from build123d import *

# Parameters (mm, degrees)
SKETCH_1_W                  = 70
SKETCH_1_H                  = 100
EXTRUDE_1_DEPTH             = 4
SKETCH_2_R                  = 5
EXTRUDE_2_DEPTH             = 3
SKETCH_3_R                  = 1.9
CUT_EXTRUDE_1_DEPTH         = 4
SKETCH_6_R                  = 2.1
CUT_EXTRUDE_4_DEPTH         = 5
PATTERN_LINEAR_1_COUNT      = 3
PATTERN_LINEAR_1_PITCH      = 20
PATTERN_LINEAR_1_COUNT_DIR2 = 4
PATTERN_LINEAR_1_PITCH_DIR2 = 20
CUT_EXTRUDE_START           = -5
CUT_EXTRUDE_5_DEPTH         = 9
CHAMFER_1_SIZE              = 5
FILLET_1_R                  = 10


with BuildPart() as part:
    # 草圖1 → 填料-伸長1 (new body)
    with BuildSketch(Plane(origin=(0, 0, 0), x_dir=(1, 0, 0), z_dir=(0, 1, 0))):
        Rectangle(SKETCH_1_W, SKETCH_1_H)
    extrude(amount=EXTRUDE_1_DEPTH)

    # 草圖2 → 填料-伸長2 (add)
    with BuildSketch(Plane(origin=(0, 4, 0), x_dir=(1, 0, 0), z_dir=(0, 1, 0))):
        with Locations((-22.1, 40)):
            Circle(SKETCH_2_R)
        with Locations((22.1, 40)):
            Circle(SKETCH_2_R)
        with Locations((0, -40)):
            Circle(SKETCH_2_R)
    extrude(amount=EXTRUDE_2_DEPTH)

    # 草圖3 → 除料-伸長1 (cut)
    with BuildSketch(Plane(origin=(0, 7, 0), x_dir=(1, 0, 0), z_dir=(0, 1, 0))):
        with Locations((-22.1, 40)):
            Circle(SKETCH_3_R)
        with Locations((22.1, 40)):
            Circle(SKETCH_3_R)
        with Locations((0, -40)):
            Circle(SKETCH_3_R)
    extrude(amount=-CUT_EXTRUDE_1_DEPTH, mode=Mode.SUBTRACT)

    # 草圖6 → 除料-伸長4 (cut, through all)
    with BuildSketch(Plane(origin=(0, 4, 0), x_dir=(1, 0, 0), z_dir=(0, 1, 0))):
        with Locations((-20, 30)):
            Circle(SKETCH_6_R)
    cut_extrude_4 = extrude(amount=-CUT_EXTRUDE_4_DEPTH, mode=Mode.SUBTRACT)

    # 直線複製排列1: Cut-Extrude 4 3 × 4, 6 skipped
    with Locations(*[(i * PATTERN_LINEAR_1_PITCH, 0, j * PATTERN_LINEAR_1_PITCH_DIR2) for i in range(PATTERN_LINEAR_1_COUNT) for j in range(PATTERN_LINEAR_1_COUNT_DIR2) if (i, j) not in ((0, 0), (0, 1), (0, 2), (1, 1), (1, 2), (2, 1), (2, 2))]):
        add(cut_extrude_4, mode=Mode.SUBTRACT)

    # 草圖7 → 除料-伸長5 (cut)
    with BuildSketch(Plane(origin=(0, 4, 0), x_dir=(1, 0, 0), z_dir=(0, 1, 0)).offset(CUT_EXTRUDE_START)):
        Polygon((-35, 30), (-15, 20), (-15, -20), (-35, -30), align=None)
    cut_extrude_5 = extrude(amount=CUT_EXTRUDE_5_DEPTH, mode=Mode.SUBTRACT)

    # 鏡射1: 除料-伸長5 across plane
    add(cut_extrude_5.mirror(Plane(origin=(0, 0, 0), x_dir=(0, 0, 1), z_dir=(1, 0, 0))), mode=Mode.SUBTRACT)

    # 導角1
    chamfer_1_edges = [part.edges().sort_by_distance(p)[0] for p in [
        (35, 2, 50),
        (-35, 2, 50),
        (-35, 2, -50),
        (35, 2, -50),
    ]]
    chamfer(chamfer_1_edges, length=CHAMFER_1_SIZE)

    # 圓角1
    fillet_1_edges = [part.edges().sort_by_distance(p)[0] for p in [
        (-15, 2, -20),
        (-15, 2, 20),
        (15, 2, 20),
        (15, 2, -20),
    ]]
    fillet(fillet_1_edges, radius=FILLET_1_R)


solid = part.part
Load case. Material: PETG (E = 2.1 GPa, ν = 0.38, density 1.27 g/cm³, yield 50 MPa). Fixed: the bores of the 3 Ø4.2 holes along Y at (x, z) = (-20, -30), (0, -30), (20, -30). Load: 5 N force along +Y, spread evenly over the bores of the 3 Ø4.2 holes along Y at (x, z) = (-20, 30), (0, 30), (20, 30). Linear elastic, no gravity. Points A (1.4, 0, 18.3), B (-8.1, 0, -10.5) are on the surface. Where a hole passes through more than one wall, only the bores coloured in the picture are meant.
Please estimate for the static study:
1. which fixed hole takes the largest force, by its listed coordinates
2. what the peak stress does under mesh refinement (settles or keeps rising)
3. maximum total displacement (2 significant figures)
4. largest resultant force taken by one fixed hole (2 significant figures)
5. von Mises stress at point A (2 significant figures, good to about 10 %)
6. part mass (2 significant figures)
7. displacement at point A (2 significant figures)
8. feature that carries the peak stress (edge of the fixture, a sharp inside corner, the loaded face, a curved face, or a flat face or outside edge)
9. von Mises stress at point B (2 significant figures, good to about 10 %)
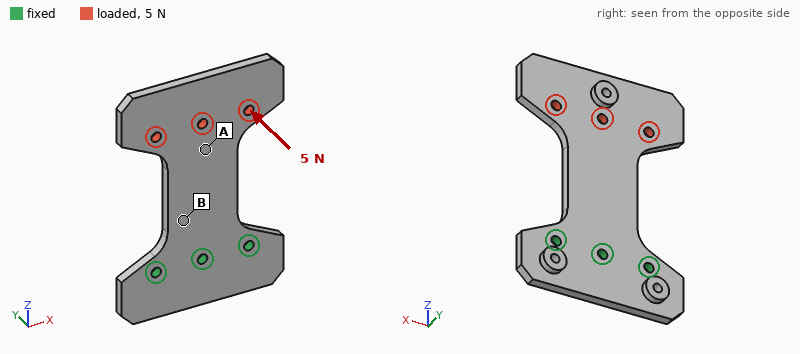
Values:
(0, -30)
keeps rising
1.4 mm
7.0 N
0.67 MPa
26 g
0.65 mm
edge of the fixture
2.4 MPa
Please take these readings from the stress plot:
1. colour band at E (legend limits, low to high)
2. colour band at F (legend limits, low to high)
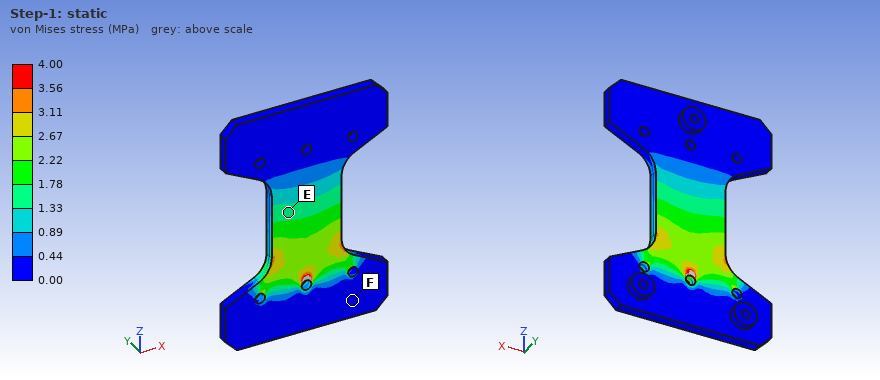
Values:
1.33 to 1.78 MPa
0.00 to 0.44 MPa
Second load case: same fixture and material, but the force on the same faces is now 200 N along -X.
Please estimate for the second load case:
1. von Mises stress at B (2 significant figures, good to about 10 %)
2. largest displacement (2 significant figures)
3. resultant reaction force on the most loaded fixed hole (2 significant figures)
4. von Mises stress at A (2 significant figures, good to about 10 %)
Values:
7.3 MPa
1.2 mm
320 N
4.2 MPa
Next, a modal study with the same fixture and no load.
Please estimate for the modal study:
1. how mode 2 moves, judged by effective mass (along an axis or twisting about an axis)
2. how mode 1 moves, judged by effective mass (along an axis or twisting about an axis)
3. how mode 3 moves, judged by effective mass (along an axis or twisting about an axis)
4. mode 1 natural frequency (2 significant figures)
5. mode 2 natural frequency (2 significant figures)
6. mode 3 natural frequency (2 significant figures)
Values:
twisting about Z
along Y
along X
97 Hz
260 Hz
660 Hz
